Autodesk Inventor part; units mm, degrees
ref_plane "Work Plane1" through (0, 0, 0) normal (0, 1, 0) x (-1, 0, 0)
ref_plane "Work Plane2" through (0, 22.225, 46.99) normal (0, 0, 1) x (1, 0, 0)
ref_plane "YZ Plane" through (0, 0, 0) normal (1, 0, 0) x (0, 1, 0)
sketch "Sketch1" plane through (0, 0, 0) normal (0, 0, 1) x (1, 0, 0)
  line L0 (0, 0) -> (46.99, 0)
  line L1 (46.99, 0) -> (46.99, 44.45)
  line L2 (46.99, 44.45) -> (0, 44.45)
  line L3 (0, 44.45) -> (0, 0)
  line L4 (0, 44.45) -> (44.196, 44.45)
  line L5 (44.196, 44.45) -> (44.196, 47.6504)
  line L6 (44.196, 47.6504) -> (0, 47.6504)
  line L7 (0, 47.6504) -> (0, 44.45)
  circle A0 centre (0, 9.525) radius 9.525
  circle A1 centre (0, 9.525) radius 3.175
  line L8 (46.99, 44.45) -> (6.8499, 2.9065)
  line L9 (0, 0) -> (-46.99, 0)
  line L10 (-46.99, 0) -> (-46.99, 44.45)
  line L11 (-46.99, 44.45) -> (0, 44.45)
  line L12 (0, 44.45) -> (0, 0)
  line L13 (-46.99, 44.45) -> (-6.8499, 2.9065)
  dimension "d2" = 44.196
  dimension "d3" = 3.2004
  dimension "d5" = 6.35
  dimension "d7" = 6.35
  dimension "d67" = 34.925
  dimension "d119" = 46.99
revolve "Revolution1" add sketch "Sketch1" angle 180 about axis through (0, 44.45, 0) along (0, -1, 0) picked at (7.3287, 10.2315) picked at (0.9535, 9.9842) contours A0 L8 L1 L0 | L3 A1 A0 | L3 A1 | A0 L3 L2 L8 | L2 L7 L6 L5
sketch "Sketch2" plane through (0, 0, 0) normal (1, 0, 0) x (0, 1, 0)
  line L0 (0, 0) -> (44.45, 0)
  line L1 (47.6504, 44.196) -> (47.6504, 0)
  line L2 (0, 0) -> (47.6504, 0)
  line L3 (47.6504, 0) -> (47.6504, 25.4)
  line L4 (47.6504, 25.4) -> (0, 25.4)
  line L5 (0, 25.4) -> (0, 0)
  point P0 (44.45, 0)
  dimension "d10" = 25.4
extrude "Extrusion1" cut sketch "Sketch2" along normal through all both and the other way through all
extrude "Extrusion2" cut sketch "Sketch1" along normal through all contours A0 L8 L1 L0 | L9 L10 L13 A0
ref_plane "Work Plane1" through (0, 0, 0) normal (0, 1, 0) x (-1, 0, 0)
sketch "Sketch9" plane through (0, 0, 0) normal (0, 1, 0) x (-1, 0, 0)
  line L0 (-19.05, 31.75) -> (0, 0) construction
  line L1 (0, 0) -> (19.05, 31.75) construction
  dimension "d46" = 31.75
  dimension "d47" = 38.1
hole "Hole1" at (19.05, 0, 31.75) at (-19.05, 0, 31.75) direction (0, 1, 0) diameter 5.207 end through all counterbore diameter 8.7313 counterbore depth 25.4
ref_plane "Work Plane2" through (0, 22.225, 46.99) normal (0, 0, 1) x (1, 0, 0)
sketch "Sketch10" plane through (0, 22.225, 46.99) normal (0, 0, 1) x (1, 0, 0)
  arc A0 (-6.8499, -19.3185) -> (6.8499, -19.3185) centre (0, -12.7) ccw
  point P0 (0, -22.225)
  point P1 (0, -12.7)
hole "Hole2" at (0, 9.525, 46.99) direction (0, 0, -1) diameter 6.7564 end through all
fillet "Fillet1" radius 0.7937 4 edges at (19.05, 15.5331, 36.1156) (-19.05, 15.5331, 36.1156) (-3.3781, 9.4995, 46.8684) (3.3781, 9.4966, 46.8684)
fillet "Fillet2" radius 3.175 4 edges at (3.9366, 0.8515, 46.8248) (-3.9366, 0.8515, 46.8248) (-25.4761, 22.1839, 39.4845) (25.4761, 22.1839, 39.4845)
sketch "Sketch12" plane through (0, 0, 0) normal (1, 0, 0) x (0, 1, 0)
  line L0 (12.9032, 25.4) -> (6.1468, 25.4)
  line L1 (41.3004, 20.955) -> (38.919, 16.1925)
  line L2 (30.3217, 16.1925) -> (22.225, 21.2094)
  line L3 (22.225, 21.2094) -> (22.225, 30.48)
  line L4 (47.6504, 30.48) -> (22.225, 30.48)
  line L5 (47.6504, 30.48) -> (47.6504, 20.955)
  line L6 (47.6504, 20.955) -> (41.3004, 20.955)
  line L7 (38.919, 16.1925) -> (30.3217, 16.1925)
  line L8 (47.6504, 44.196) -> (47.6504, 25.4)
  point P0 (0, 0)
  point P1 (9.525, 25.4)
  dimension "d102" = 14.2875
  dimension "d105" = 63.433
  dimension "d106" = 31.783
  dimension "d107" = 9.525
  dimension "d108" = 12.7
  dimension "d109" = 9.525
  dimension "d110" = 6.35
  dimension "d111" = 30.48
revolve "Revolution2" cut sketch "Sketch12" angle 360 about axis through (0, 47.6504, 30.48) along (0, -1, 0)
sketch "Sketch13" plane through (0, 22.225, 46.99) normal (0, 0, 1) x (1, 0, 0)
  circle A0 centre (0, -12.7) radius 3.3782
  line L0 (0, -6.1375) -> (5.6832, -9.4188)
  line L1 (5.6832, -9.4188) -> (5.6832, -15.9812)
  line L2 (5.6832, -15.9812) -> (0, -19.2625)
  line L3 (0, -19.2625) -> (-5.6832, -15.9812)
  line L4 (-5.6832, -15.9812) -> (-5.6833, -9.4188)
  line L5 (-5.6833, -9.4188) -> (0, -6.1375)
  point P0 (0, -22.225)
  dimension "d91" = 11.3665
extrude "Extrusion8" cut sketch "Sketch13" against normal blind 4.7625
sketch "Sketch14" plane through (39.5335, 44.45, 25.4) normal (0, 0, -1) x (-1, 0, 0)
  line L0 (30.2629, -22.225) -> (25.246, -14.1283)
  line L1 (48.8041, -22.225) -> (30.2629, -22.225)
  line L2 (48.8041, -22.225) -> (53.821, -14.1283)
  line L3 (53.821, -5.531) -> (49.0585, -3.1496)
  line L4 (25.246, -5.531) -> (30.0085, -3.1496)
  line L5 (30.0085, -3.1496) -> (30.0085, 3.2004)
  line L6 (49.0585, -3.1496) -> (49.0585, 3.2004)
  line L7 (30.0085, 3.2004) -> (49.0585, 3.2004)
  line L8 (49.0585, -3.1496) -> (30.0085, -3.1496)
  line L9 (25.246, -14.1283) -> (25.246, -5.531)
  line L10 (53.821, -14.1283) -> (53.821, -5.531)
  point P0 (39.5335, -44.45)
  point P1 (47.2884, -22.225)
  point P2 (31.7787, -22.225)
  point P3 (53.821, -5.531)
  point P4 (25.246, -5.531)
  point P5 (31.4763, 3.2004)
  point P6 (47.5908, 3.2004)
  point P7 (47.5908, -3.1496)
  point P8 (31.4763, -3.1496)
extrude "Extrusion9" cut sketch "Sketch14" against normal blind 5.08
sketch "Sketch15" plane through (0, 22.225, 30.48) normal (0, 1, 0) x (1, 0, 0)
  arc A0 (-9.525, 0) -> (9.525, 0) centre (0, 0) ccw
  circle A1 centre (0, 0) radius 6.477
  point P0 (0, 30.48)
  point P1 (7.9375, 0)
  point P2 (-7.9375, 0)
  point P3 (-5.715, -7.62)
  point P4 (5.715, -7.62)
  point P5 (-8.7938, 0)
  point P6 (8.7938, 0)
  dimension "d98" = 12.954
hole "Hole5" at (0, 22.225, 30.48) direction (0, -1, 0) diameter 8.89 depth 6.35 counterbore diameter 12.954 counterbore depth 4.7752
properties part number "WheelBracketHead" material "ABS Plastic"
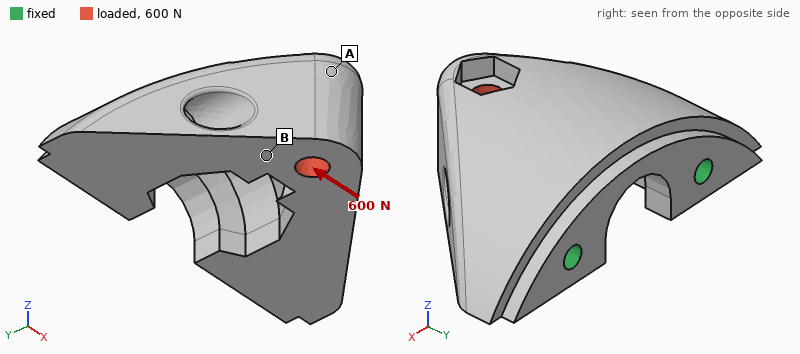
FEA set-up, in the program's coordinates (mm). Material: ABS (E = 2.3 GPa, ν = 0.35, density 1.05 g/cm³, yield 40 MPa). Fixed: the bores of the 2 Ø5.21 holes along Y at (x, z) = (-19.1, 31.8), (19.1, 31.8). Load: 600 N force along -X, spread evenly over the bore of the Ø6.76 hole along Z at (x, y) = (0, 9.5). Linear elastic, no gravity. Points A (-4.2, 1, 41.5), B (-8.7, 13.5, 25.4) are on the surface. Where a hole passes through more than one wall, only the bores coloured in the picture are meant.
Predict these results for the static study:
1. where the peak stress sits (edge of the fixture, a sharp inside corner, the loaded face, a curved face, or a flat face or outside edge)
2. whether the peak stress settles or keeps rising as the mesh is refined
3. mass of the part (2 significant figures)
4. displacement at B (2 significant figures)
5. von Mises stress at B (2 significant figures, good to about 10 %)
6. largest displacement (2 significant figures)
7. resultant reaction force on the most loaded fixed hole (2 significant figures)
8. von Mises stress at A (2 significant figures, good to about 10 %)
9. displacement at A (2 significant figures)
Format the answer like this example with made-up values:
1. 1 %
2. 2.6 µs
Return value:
1. edge of the fixture
2. keeps rising
3. 30 g
4. 53 µm
5. 2.3 MPa
6. 74 µm
7. 410 N
8. 1.0 MPa
9. 47 µm
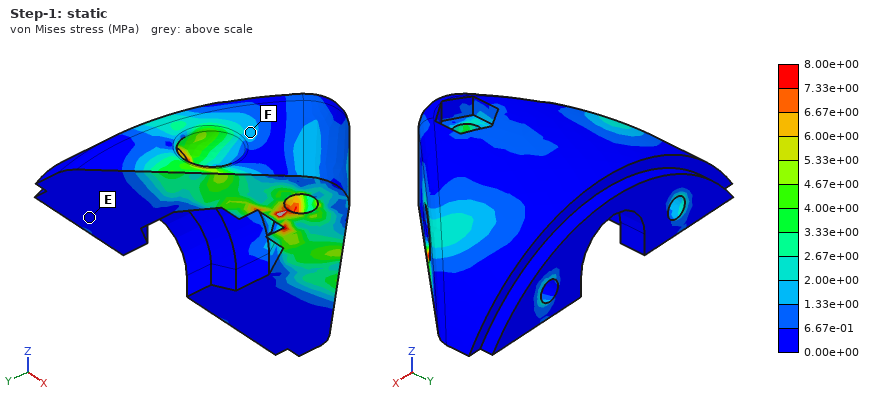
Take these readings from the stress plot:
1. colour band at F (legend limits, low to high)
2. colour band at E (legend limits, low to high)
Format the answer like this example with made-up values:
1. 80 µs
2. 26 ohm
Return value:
1. 1.33e+00 to 2.00e+00 MPa
2. 0.00e+00 to 6.67e-01 MPa
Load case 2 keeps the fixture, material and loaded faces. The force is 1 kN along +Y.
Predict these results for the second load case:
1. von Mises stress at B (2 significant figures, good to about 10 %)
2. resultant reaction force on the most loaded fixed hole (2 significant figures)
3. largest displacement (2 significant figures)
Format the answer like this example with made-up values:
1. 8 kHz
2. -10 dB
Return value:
1. 3.5 MPa
2. 550 N
3. 80 µm
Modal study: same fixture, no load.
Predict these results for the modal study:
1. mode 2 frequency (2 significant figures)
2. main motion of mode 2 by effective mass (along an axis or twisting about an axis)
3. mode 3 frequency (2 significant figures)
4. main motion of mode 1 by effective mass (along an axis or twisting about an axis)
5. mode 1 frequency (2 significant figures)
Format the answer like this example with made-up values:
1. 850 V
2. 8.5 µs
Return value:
1. 5700 Hz
2. along X
3. 7500 Hz
4. along Z
5. 3100 Hz
